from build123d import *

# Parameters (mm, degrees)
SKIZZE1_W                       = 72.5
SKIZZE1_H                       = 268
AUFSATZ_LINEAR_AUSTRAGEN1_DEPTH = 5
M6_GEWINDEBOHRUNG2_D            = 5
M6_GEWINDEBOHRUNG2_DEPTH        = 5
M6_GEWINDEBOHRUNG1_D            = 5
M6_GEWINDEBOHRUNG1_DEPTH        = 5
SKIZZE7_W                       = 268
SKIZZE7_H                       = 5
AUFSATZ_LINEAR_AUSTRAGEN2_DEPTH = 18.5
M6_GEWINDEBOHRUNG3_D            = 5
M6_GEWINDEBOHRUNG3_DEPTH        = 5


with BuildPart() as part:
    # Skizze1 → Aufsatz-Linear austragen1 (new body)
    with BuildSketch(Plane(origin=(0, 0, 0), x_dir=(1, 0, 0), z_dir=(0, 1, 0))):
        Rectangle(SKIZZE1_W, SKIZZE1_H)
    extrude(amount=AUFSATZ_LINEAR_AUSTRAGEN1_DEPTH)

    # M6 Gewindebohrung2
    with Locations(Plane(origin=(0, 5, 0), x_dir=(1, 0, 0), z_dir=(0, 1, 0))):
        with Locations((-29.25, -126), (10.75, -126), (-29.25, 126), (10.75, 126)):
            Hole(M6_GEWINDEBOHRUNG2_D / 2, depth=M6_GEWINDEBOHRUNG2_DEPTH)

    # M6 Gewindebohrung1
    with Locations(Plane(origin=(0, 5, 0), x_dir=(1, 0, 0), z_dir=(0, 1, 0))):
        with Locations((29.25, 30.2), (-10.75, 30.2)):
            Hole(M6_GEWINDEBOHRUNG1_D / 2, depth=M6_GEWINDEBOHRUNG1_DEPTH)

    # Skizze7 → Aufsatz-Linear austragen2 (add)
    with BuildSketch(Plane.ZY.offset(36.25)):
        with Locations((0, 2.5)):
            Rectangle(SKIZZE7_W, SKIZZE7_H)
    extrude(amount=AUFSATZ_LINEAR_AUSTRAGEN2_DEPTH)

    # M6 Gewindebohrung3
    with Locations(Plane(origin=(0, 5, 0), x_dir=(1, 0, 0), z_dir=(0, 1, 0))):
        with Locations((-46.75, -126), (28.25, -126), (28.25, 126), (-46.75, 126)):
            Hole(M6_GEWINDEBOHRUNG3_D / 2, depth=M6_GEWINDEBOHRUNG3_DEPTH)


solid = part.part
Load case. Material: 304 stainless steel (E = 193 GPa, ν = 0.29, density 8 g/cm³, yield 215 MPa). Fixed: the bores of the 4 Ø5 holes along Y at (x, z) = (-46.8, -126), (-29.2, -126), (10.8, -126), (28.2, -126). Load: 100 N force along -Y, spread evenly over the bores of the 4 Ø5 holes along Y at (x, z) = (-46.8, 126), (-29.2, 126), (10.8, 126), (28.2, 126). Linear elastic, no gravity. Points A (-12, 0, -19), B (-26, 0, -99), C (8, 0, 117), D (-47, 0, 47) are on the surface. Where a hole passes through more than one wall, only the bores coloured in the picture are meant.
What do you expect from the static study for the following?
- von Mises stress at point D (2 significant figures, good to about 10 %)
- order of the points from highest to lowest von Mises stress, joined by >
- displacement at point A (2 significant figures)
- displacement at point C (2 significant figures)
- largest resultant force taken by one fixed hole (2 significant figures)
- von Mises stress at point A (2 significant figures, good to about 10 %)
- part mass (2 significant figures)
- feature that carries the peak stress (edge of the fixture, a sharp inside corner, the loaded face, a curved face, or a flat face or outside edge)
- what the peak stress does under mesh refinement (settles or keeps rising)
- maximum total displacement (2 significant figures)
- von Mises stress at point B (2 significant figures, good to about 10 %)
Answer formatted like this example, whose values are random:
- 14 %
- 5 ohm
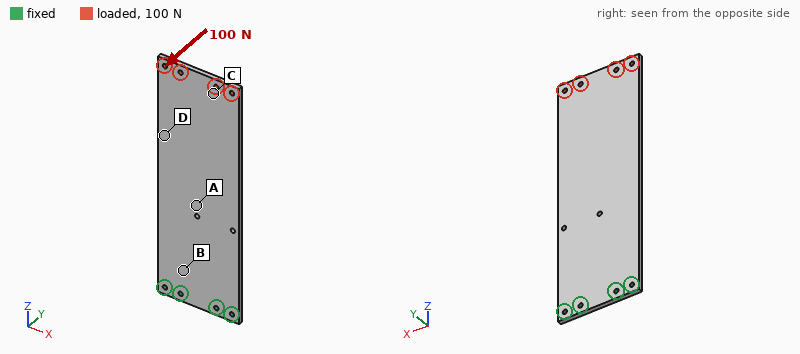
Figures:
- 21 MPa
- B > A > D > C
- 0.68 mm
- 2.7 mm
- 130 N
- 36 MPa
- 970 g
- edge of the fixture
- keeps rising
- 3.0 mm
- 54 MPa
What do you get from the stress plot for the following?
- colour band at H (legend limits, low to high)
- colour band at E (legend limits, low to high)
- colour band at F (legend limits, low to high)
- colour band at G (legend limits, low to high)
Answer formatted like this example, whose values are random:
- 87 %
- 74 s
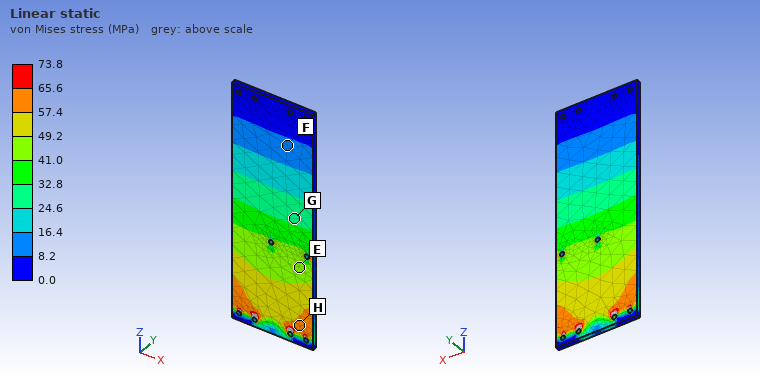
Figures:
- 57.4 to 65.6 MPa
- 41.0 to 49.2 MPa
- 8.2 to 16.4 MPa
- 24.6 to 32.8 MPa
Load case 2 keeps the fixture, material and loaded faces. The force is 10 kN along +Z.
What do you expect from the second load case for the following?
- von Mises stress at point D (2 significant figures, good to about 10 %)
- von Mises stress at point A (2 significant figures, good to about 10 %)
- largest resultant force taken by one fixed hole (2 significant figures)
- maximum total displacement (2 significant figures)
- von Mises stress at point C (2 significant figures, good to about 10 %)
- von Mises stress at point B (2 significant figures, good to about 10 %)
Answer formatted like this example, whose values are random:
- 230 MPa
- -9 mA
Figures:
- 22 MPa
- 19 MPa
- 2.8 kN
- 32 µm
- 27 MPa
- 22 MPa
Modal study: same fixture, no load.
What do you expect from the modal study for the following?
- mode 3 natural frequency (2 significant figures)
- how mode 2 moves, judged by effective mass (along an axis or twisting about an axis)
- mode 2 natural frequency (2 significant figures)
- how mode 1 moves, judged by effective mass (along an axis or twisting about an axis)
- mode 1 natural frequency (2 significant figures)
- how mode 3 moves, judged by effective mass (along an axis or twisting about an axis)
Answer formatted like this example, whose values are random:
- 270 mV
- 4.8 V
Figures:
- 370 Hz
- twisting about Z
- 350 Hz
- along Y
- 59 Hz
- along Y
